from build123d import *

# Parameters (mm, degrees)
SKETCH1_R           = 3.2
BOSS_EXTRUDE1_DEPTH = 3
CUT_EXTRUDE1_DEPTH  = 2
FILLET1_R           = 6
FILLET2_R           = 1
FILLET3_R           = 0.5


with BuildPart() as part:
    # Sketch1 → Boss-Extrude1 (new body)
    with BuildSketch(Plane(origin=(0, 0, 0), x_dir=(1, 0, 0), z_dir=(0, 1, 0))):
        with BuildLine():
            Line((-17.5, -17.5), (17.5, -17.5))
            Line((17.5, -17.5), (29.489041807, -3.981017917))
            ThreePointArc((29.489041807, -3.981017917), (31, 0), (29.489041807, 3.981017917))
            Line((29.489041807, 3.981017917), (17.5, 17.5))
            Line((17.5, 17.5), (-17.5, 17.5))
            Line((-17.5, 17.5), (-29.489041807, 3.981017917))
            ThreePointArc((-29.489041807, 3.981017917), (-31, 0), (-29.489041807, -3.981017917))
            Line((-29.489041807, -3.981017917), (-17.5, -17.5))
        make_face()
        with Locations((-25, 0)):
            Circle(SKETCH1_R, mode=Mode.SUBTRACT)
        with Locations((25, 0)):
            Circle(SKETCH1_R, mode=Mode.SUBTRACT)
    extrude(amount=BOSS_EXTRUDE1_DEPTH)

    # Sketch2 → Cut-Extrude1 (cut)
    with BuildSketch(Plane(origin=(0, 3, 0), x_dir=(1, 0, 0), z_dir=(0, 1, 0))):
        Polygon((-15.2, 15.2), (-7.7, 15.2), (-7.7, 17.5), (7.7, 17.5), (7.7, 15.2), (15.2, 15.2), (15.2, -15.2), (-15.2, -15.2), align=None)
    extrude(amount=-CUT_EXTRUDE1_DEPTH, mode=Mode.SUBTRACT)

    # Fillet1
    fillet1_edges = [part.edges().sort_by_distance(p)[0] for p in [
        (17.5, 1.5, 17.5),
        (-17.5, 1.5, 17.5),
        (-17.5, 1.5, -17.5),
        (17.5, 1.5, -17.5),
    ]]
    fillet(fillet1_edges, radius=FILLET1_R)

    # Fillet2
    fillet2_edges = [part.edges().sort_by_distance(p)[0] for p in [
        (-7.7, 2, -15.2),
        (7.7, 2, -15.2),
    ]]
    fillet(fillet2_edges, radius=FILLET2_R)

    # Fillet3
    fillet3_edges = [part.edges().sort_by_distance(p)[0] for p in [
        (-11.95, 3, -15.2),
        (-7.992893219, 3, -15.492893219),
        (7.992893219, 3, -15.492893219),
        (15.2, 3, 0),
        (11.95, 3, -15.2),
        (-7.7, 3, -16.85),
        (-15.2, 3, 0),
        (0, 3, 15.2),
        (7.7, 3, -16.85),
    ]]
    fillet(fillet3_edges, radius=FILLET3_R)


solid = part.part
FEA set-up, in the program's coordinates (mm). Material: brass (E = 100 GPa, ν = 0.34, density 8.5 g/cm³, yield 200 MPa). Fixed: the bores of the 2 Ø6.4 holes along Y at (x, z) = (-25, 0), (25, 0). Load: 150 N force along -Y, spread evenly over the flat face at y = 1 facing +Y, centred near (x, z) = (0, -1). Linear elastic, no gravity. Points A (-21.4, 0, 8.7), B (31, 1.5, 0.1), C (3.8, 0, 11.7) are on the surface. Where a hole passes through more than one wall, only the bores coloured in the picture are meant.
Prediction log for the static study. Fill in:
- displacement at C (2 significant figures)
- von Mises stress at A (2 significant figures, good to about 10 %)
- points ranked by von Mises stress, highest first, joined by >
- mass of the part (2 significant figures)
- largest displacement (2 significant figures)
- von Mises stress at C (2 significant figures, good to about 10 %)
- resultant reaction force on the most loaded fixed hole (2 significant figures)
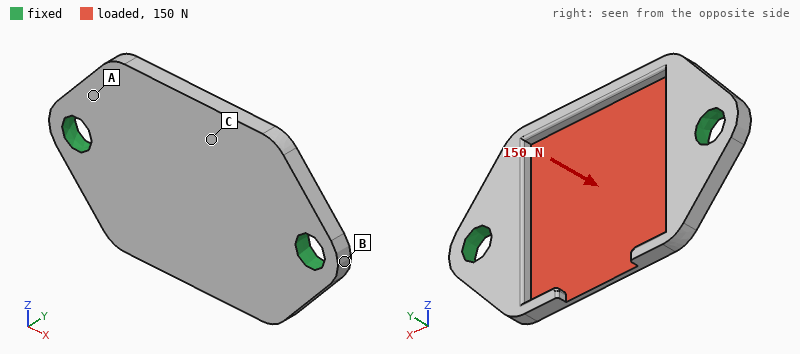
26 µm
11 MPa
C > A > B
27 g
44 µm
19 MPa
140 N
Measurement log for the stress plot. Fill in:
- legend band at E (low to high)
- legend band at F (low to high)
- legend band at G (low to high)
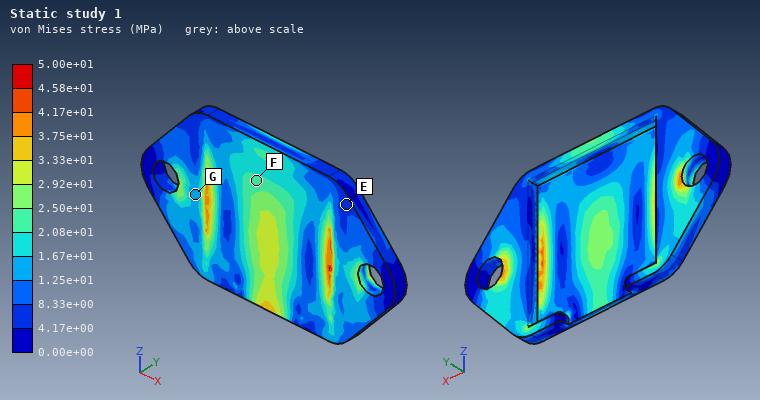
4.17e+00 to 8.33e+00 MPa
2.08e+01 to 2.50e+01 MPa
1.25e+01 to 1.67e+01 MPa
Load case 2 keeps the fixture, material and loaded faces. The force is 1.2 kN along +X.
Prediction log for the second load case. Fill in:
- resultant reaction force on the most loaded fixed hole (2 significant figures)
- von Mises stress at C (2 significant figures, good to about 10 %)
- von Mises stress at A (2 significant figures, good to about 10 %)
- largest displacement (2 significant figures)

600 N
3.9 MPa
14 MPa
9.7 µm
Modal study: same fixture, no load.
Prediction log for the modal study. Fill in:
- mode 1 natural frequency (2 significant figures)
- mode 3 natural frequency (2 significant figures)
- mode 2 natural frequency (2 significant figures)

3600 Hz
5900 Hz
3600 Hz
